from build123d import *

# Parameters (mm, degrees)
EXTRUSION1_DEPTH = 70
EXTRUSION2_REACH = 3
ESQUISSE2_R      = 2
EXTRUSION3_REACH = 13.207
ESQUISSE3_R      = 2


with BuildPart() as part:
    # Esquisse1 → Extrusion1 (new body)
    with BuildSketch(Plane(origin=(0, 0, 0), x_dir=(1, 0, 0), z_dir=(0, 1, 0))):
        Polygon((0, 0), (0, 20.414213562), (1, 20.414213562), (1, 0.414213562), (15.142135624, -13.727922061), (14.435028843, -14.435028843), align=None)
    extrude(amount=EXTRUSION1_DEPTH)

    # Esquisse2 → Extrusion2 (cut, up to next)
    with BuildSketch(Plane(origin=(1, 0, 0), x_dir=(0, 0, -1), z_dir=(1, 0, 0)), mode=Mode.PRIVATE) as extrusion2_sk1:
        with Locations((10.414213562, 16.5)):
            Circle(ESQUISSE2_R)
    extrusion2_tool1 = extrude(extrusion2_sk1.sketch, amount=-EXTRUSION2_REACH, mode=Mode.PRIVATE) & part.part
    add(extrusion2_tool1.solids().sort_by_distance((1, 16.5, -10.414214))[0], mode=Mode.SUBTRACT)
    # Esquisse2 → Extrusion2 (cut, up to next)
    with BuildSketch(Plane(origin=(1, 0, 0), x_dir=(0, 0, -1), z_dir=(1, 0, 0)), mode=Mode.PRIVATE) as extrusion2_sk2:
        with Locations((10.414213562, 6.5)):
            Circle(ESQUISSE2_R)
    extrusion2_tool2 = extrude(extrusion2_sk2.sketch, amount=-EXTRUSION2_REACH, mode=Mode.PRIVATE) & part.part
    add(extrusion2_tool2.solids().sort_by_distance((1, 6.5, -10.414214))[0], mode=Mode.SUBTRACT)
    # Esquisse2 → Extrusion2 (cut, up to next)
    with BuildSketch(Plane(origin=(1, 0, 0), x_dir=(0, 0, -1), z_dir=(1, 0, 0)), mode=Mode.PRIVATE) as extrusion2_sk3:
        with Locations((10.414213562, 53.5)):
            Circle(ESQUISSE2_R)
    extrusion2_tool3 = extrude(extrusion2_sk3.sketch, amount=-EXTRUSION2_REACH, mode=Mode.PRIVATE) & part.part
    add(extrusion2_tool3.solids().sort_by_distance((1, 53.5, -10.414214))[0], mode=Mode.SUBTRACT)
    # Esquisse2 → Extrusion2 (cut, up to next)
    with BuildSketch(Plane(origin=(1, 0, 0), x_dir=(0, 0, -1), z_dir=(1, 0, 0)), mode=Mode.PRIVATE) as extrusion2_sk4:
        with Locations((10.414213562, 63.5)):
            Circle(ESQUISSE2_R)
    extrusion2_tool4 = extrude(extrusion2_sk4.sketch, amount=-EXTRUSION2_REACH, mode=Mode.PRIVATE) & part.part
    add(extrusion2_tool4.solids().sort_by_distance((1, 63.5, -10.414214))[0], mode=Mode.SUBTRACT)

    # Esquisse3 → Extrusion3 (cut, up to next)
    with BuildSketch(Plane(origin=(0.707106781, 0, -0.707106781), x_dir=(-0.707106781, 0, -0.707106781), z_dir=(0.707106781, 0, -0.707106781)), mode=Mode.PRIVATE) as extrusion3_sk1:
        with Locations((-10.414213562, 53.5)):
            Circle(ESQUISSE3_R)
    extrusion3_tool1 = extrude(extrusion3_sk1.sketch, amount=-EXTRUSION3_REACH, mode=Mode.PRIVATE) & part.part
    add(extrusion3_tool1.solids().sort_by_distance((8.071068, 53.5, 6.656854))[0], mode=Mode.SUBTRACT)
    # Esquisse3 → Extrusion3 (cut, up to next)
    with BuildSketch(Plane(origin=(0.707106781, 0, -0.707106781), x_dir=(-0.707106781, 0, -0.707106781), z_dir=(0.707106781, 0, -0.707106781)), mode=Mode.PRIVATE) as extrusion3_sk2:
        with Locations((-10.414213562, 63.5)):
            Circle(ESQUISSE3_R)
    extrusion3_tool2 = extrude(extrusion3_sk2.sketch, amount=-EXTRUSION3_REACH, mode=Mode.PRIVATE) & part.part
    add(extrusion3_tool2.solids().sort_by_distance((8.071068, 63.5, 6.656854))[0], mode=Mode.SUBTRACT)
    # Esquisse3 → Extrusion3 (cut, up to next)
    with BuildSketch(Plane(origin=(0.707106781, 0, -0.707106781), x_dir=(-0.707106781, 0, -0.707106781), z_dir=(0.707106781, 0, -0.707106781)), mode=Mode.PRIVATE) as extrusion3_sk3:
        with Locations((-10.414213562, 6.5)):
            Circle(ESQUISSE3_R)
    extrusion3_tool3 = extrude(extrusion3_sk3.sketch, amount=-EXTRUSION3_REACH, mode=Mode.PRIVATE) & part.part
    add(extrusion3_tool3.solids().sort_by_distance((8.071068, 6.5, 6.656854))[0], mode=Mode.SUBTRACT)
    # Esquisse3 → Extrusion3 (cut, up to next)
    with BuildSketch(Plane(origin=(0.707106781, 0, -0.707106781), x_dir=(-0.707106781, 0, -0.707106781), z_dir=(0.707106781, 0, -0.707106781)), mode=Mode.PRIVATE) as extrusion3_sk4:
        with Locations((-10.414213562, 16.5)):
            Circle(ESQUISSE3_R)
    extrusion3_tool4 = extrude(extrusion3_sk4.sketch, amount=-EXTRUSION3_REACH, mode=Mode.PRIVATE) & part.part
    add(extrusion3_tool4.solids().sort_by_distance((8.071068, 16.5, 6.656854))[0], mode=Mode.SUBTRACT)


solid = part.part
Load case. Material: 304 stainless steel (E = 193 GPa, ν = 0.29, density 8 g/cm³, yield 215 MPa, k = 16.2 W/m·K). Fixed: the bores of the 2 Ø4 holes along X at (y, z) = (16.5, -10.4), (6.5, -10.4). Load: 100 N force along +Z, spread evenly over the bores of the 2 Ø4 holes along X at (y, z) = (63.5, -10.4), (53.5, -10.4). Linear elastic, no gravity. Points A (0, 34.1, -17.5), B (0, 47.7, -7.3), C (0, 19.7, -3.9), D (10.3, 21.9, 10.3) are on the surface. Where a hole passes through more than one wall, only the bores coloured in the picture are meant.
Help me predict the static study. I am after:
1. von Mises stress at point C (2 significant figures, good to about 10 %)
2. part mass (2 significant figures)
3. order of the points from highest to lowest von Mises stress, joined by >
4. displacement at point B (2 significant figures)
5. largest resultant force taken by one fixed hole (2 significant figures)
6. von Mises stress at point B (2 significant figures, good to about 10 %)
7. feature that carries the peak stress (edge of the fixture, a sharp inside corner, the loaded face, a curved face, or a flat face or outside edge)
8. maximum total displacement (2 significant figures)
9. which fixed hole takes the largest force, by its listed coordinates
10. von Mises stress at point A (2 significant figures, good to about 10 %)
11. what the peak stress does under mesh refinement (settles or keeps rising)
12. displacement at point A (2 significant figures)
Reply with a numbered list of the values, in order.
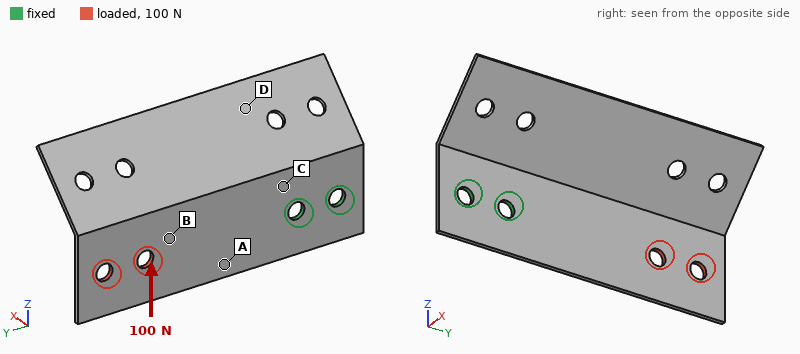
1. 26 MPa
2. 22 g
3. C > A > B > D
4. 26 µm
5. 370 N
6. 11 MPa
7. edge of the fixture
8. 53 µm
9. (16.5, -10.4)
10. 18 MPa
11. keeps rising
12. 11 µm
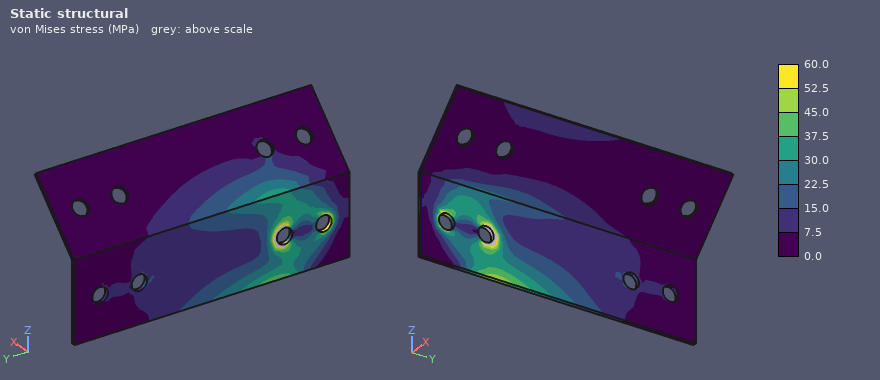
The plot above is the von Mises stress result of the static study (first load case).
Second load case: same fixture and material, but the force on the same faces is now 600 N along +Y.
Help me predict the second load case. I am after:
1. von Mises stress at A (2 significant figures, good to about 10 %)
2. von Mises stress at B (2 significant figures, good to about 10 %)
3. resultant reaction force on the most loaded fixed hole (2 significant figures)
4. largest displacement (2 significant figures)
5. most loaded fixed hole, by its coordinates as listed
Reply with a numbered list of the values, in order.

1. 34 MPa
2. 30 MPa
3. 460 N
4. 11 µm
5. (16.5, -10.4)
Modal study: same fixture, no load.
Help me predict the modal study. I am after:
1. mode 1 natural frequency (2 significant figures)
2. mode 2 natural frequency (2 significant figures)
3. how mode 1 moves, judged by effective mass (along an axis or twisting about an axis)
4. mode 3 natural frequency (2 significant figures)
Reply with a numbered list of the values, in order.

1. 460 Hz
2. 720 Hz
3. along X
4. 1300 Hz
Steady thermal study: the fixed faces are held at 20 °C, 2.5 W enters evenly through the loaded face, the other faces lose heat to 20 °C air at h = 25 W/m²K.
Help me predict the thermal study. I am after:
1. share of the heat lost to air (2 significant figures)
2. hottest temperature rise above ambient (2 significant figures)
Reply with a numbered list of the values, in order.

1. 92 %
2. 70 K
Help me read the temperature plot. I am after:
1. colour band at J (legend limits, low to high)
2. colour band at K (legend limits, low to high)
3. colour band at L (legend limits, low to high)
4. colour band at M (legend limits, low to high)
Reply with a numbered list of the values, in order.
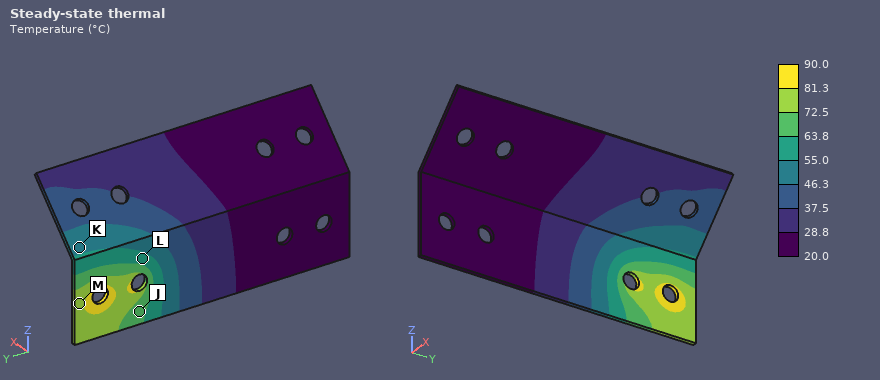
1. 63.8 to 72.5 °C
2. 46.3 to 55.0 °C
3. 55.0 to 63.8 °C
4. 72.5 to 81.3 °C
